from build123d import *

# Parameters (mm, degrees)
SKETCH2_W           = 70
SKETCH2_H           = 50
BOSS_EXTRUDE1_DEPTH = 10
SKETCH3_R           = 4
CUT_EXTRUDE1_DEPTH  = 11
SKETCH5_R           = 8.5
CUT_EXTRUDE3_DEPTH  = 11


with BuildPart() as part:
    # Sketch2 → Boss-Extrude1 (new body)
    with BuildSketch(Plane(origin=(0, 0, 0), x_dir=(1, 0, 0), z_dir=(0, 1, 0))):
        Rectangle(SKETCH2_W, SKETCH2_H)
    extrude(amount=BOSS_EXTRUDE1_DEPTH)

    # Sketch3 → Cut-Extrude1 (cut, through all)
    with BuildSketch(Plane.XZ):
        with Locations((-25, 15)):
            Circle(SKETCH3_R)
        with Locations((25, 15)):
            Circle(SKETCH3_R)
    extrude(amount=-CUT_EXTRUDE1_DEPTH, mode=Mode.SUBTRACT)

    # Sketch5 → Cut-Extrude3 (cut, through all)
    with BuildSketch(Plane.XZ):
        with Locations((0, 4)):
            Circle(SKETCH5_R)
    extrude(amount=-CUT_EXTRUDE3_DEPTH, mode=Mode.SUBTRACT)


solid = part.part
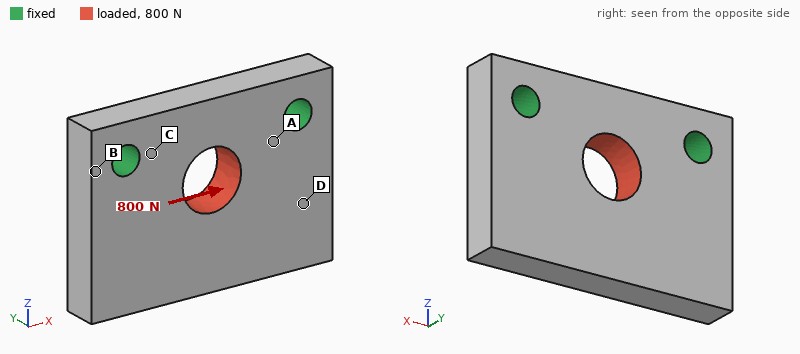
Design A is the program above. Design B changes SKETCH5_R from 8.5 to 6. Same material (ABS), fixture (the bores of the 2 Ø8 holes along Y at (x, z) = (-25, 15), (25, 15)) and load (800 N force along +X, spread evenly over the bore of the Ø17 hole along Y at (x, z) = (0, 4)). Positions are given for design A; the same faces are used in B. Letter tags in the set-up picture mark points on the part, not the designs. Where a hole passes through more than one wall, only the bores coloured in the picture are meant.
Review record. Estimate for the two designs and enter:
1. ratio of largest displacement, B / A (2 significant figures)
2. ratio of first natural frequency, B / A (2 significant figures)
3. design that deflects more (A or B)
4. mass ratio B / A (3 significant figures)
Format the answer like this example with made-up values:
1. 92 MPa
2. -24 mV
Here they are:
1. 0.90
2. 1.0
3. A
4. 1.04
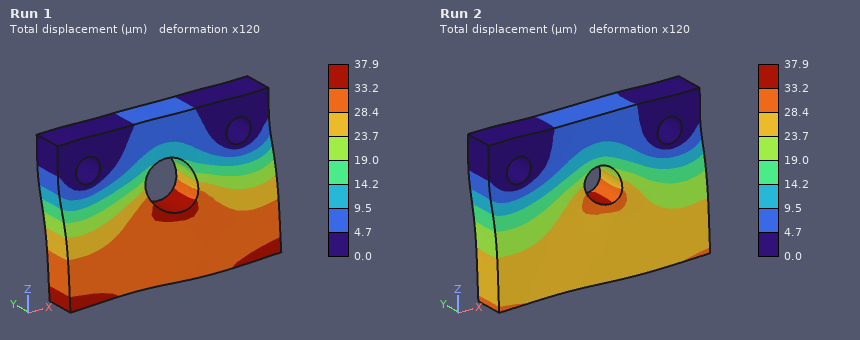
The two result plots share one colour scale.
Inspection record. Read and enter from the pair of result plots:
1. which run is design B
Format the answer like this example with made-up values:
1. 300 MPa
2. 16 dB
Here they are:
1. Run 2
